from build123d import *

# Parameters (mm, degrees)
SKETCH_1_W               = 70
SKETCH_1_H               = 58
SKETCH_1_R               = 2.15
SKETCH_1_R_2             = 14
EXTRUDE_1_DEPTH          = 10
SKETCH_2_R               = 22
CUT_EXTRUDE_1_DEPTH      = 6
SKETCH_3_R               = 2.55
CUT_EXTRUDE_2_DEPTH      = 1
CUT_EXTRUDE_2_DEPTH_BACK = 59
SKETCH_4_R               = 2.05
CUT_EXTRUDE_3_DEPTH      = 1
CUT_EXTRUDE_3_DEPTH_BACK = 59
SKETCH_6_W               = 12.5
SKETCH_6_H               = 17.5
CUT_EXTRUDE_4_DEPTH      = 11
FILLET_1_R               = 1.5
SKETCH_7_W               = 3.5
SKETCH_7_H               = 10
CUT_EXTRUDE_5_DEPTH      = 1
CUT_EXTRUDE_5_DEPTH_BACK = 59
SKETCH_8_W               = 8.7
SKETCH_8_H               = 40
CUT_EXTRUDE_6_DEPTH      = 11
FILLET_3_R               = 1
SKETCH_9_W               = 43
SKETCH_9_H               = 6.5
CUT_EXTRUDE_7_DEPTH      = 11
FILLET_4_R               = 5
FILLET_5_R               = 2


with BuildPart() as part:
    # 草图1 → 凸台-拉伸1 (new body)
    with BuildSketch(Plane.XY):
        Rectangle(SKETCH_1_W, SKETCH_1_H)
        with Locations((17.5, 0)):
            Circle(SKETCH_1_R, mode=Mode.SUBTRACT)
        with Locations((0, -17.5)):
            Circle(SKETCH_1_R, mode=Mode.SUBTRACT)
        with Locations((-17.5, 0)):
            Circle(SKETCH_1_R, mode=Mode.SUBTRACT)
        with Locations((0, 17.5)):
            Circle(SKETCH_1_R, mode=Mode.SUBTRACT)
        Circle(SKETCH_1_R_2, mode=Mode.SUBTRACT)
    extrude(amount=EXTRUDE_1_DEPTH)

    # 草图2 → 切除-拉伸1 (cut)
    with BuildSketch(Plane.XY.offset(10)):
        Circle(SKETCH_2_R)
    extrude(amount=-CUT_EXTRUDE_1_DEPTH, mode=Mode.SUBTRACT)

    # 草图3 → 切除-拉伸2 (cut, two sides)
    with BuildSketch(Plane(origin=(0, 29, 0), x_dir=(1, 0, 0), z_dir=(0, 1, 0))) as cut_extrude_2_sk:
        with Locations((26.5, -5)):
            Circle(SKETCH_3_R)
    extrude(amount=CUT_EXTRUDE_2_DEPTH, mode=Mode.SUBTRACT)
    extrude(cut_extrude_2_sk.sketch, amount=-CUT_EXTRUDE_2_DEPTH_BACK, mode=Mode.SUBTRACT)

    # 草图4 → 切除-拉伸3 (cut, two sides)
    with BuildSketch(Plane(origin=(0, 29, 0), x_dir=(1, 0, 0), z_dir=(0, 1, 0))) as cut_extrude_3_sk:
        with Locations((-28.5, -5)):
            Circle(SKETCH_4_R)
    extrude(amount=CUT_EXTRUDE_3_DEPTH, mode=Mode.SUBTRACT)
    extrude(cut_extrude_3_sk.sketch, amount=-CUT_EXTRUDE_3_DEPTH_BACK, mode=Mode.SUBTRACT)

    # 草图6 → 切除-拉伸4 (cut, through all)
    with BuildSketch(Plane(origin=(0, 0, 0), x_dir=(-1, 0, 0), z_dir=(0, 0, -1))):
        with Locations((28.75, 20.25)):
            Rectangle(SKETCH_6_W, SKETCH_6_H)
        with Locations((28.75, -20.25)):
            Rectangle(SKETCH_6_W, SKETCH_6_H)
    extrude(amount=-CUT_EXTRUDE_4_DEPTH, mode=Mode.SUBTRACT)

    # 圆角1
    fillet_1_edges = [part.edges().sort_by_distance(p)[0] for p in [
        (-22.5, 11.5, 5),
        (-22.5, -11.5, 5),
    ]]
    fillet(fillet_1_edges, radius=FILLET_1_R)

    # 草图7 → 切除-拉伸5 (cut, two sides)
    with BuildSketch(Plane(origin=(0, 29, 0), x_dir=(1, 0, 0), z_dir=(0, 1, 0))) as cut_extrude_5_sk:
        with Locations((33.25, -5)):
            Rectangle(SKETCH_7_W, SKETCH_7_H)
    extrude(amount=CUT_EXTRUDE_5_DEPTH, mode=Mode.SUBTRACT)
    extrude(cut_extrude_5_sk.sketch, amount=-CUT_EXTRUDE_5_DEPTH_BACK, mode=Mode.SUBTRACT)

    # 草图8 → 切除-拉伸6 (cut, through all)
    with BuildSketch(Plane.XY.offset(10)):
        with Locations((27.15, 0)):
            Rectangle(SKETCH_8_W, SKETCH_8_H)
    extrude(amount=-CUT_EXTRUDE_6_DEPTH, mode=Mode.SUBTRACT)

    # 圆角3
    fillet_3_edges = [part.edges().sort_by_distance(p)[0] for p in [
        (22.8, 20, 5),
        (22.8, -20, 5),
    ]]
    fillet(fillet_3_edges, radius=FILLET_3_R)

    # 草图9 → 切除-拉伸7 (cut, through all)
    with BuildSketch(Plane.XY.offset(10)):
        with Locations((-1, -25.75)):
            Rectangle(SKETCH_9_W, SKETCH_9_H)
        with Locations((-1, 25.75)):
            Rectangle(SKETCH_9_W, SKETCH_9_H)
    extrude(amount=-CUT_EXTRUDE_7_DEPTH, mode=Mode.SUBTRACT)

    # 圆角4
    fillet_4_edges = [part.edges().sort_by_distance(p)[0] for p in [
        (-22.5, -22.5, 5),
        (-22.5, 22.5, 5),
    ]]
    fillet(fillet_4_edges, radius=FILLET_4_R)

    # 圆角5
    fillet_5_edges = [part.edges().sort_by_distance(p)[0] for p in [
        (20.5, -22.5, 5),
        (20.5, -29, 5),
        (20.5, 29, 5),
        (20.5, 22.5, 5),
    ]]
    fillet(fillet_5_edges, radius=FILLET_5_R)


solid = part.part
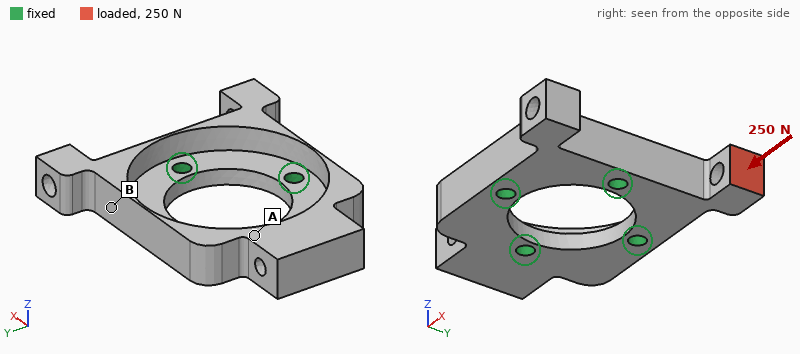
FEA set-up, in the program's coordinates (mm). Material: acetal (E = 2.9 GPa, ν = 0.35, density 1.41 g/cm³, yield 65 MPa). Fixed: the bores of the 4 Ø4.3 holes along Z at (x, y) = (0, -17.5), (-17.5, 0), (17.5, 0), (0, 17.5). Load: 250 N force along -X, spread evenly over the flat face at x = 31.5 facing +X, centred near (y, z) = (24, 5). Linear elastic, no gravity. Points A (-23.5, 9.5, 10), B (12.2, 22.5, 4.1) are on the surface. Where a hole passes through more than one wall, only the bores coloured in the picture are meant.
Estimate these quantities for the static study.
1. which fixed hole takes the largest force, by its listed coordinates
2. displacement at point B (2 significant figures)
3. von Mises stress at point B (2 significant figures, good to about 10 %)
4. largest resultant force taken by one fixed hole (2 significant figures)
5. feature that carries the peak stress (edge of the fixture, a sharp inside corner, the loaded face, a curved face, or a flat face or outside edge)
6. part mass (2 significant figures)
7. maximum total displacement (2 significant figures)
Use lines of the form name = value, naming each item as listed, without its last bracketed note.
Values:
which fixed hole takes the largest force, by its listed coordinates = (0, 17.5)
displacement at point B = 0.10 mm
von Mises stress at point B = 12 MPa
largest resultant force taken by one fixed hole = 280 N
feature that carries the peak stress = a curved face
part mass = 18 g
maximum total displacement = 0.45 mm
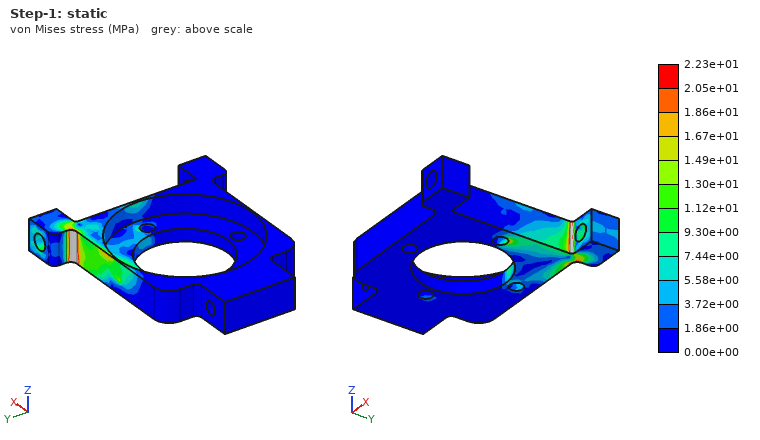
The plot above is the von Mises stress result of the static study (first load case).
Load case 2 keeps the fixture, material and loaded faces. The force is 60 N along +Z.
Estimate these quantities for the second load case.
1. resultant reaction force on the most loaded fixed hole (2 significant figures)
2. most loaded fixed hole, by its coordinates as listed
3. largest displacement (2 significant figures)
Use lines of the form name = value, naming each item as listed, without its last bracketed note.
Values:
resultant reaction force on the most loaded fixed hole = 61 N
most loaded fixed hole, by its coordinates as listed = (17.5, 0)
largest displacement = 0.93 mm
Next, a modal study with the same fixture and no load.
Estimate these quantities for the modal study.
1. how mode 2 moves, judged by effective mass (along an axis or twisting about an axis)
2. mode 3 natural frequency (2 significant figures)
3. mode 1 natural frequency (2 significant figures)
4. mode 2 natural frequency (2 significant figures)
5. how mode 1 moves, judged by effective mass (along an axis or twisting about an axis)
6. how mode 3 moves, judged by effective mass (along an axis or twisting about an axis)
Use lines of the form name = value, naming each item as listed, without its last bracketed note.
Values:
how mode 2 moves, judged by effective mass = along Z
mode 3 natural frequency = 2600 Hz
mode 1 natural frequency = 1300 Hz
mode 2 natural frequency = 1600 Hz
how mode 1 moves, judged by effective mass = twisting about X
how mode 3 moves, judged by effective mass = along Z
